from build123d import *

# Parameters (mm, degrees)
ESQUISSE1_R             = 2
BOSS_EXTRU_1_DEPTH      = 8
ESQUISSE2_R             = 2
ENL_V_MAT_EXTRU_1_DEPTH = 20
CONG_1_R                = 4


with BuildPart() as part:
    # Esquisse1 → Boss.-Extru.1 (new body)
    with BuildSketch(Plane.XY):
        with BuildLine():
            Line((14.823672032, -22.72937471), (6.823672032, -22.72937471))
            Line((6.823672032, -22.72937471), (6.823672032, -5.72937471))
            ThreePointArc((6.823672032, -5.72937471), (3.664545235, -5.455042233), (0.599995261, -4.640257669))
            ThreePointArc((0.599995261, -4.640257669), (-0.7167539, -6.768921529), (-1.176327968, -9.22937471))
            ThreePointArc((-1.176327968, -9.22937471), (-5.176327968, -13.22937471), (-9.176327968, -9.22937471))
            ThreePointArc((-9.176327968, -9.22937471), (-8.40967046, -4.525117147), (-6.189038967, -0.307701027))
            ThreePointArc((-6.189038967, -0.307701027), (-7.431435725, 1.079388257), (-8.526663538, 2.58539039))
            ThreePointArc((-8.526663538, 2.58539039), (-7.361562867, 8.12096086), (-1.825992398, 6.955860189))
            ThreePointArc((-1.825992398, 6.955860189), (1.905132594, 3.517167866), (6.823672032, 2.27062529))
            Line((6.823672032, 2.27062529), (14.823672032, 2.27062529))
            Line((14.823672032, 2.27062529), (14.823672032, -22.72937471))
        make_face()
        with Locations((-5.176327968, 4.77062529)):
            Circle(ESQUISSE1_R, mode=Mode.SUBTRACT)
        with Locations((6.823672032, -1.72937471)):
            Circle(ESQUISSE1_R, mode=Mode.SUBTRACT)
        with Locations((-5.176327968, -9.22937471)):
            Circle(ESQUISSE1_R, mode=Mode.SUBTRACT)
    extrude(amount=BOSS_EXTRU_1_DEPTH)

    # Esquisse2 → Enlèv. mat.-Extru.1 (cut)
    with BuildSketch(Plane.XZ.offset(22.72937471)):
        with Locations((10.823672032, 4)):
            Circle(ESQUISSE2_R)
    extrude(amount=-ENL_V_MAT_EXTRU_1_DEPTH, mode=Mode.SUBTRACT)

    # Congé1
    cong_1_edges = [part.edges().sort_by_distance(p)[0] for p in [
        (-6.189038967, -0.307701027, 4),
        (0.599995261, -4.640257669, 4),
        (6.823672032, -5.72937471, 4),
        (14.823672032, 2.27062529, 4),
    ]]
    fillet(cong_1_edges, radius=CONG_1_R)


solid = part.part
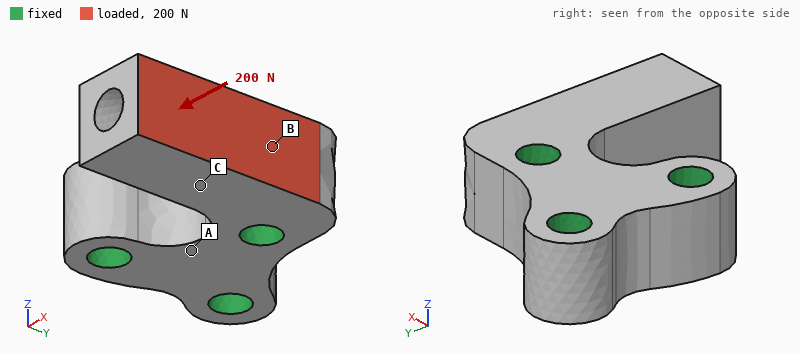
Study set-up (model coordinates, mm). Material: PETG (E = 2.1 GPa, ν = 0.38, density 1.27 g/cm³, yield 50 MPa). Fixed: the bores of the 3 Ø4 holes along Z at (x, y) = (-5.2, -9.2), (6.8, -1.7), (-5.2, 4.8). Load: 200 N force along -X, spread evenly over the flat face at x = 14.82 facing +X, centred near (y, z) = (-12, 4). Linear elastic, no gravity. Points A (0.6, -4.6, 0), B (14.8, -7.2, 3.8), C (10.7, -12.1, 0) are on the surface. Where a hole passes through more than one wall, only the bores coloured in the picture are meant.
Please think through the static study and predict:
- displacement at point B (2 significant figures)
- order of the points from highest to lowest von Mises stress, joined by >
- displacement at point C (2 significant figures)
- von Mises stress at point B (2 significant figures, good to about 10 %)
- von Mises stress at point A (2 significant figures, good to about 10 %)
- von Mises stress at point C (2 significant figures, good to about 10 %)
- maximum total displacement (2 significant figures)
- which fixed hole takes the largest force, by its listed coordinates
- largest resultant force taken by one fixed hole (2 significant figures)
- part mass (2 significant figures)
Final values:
0.13 mm
B > C > A
0.17 mm
12 MPa
3.0 MPa
7.1 MPa
0.44 mm
(6.8, -1.7)
180 N
3.6 g
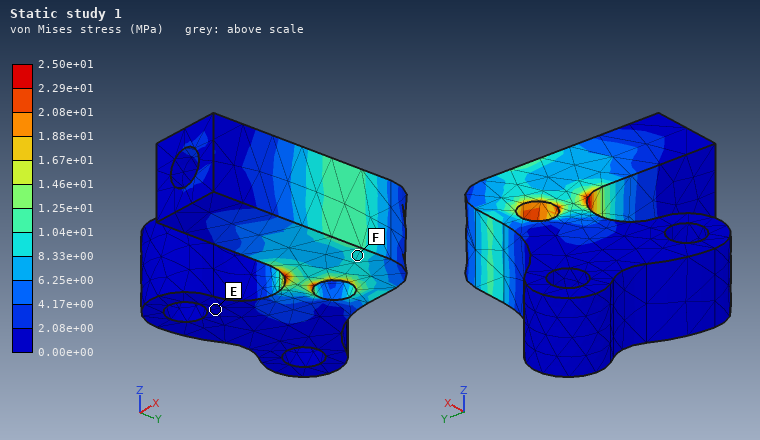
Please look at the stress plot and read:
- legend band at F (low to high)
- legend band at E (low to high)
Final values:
8.33e+00 to 1.04e+01 MPa
0.00e+00 to 2.08e+00 MPa
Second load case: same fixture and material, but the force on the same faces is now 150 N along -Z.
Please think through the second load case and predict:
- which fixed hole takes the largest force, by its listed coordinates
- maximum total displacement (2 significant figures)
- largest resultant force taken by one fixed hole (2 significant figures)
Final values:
(6.8, -1.7)
0.38 mm
160 N
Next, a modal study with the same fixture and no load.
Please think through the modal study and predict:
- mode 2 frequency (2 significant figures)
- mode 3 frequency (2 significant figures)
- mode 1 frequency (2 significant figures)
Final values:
3700 Hz
8800 Hz
3600 Hz
